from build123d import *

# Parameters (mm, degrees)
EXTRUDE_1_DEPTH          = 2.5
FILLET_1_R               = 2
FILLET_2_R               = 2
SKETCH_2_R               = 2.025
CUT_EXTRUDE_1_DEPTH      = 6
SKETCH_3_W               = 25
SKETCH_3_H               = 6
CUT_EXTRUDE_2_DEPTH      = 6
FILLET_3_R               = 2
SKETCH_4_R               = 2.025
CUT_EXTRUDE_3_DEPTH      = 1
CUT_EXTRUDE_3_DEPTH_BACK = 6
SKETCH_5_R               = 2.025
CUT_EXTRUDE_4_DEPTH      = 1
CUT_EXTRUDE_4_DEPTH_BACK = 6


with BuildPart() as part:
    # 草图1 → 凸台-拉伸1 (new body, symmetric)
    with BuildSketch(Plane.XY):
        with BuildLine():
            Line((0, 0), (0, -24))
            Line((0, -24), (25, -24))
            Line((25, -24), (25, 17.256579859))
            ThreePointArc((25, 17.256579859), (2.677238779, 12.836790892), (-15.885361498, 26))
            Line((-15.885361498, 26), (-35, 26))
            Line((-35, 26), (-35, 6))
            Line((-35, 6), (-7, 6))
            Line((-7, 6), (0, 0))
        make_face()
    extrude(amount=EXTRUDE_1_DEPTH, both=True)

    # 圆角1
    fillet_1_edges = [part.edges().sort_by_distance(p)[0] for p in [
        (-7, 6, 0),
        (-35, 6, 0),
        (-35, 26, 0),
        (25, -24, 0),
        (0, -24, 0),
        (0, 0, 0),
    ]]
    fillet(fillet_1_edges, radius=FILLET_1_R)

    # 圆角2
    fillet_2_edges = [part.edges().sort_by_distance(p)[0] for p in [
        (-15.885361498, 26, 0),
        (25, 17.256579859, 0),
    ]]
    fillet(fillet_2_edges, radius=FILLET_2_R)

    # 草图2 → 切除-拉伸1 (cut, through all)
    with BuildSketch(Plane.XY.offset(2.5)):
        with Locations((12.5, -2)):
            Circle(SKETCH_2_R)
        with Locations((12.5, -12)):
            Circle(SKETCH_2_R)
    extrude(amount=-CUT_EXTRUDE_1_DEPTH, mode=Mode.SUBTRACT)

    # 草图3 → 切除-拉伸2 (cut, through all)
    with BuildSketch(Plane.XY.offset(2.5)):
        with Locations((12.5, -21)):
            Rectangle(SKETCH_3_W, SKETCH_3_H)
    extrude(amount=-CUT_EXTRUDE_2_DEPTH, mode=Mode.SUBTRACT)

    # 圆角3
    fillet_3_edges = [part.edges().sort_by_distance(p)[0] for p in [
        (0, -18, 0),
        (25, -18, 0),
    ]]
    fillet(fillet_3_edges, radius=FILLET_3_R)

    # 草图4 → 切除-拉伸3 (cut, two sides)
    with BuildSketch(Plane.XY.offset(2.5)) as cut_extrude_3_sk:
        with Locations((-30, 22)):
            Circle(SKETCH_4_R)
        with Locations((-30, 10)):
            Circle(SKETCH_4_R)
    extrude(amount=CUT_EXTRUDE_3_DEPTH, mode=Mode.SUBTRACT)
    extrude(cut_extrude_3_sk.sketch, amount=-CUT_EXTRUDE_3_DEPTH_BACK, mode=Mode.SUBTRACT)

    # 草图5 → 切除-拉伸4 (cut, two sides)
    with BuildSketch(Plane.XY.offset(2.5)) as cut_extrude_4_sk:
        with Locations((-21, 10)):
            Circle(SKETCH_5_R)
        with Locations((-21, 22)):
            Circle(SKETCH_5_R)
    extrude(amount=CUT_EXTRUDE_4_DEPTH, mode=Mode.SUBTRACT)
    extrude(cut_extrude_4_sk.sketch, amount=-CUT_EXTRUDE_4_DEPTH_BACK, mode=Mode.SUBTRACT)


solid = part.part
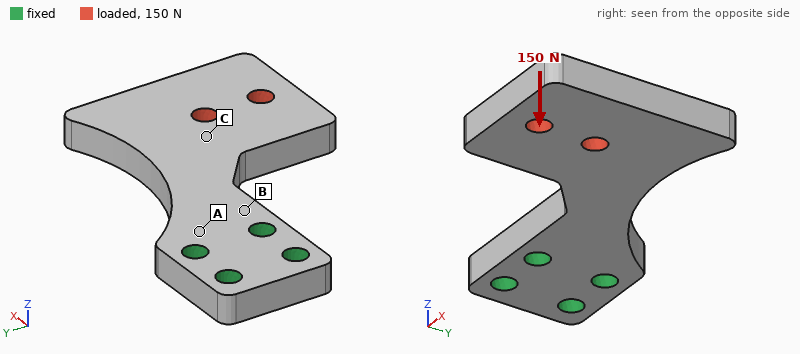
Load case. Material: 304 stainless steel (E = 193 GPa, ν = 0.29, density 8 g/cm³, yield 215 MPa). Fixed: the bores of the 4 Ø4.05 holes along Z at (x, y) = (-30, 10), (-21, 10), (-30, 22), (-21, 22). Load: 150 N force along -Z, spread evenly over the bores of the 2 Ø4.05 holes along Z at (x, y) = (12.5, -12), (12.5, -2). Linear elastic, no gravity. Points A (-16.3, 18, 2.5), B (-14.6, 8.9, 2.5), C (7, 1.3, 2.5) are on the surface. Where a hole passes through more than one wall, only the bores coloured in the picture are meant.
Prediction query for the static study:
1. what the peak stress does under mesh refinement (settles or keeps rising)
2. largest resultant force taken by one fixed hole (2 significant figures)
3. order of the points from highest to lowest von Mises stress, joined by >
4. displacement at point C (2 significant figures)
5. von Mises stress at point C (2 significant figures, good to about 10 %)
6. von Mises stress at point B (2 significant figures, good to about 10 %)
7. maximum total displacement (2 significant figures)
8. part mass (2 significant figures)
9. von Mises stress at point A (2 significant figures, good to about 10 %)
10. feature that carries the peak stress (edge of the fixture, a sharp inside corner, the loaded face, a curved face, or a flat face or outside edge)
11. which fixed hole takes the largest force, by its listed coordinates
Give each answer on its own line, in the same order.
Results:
keeps rising
340 N
B > A > C
0.071 mm
19 MPa
90 MPa
0.18 mm
52 g
47 MPa
edge of the fixture
(-21, 10)
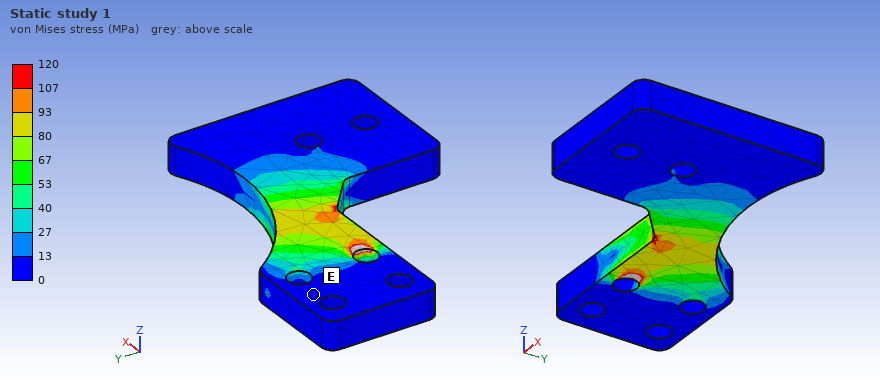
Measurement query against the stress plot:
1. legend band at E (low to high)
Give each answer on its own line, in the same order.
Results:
0 to 13 MPa
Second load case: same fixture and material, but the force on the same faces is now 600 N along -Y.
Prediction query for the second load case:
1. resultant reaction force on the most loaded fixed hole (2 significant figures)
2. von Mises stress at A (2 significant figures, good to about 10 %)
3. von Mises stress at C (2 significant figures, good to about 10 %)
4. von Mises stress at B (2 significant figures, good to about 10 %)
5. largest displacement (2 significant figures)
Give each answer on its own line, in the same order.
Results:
1.5 kN
42 MPa
19 MPa
56 MPa
94 µm
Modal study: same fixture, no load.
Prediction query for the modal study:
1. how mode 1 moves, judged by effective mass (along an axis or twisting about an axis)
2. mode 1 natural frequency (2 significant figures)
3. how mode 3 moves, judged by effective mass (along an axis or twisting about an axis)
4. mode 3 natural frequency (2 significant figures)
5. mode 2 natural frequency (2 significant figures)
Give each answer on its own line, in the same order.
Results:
along Z
1100 Hz
twisting about X
3200 Hz
2500 Hz
